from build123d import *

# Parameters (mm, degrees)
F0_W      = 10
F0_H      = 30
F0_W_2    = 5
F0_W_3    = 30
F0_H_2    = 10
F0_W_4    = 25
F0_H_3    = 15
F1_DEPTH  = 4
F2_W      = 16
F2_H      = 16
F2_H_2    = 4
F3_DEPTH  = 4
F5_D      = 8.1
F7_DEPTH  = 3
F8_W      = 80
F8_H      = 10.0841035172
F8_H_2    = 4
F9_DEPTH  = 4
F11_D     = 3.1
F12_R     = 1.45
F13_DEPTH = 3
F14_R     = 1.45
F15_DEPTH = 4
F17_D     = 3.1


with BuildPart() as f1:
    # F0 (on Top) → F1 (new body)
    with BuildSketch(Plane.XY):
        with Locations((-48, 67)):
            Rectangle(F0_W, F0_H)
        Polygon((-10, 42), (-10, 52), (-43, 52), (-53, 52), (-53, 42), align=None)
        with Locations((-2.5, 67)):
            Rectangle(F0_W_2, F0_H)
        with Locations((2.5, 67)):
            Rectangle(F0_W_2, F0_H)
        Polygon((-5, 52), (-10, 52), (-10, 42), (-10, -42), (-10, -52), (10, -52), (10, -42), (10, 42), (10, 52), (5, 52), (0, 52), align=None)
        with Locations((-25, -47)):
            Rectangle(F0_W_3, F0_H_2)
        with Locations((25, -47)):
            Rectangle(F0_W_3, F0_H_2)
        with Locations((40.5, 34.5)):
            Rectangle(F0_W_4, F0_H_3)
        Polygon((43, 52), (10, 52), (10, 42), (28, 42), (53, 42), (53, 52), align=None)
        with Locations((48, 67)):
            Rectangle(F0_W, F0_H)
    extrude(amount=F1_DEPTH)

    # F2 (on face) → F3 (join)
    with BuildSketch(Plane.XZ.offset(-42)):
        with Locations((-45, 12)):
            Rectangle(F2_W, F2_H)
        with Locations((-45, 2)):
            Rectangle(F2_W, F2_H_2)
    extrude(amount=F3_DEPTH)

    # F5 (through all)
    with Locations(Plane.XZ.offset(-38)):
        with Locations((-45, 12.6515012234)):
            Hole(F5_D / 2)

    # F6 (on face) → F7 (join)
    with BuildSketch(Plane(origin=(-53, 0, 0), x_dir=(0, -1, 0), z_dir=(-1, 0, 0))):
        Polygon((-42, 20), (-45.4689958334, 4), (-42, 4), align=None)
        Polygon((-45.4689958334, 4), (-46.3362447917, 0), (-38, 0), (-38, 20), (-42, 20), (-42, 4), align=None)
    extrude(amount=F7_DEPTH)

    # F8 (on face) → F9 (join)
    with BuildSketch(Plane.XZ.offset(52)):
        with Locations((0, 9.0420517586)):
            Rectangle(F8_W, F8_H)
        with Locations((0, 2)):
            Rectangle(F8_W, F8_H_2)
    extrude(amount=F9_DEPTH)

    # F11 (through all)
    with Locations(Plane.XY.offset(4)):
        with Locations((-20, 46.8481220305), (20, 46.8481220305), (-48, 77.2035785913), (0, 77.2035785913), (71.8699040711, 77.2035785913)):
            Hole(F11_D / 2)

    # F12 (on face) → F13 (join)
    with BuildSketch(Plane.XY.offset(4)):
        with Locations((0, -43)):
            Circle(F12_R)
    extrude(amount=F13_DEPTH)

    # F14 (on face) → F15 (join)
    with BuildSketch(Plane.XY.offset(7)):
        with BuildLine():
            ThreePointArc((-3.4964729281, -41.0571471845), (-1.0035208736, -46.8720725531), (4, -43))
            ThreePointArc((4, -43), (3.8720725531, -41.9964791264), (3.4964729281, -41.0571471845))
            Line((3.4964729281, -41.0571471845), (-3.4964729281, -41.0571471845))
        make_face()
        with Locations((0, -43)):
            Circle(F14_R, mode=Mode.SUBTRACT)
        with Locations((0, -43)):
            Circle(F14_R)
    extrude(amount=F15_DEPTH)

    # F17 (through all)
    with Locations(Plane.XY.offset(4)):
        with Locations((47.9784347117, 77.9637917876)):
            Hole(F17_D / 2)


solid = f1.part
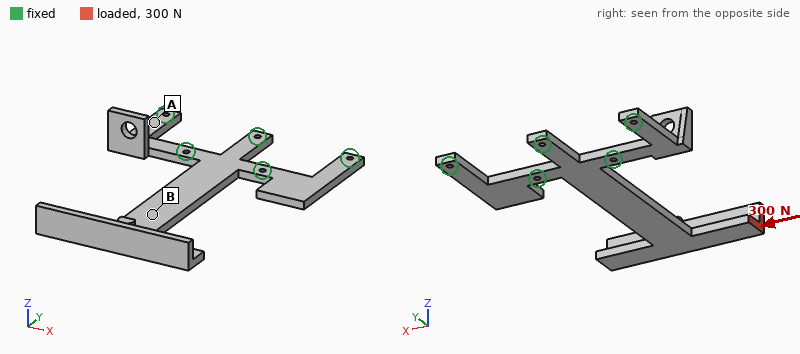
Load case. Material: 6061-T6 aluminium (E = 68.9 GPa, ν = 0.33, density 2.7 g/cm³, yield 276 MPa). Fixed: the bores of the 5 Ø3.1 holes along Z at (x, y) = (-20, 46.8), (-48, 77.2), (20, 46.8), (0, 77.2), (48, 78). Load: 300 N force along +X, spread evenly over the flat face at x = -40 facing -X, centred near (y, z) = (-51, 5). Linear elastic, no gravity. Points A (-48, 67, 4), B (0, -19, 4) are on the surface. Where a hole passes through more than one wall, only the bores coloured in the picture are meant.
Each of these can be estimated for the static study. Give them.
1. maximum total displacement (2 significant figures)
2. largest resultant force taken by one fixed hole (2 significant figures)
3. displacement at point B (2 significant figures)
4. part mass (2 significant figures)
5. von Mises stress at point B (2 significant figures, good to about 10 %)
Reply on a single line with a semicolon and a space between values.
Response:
0.89 mm; 840 N; 0.35 mm; 68 g; 26 MPa
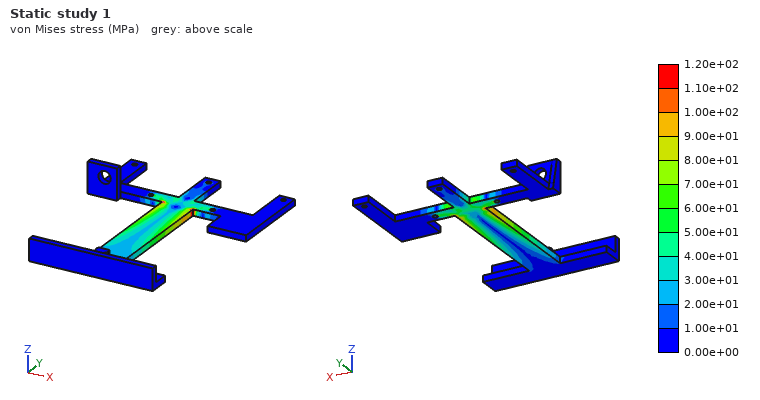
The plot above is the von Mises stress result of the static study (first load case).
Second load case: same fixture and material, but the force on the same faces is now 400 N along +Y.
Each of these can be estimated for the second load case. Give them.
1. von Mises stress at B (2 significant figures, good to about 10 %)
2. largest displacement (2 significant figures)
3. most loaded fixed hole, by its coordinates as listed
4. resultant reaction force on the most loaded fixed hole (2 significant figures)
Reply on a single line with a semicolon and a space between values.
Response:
26 MPa; 1.3 mm; (-20, 46.8); 540 N
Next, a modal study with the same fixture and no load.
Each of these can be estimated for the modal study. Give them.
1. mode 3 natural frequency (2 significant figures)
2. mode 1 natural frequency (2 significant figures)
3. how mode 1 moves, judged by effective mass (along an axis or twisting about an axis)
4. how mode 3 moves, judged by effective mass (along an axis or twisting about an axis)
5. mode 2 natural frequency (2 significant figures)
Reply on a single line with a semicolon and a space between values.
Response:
690 Hz; 140 Hz; along Z; along X; 480 Hz
